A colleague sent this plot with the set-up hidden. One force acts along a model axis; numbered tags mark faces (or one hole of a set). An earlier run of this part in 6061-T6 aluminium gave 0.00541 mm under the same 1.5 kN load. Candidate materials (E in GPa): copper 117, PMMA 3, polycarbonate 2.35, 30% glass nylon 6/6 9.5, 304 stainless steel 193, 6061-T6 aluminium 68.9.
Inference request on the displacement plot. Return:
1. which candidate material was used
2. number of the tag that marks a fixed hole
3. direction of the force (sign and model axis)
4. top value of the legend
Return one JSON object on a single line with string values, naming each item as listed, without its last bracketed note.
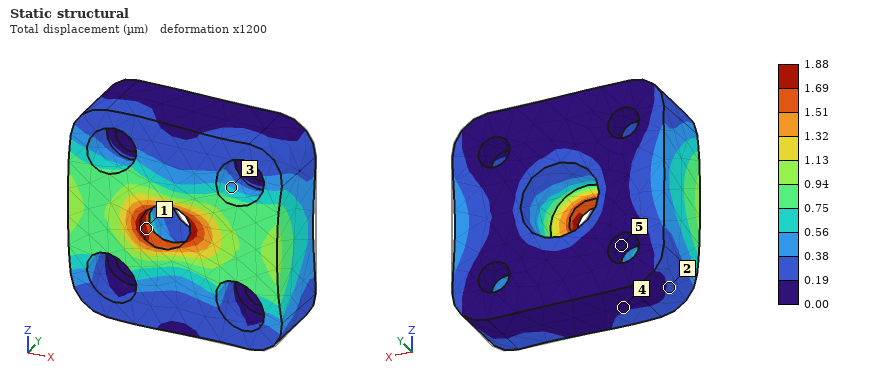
{"which candidate material was used": "304 stainless steel", "number of the tag that marks a fixed hole": "5", "direction of the force": "-X", "top value of the legend": "1.88 µm"}
